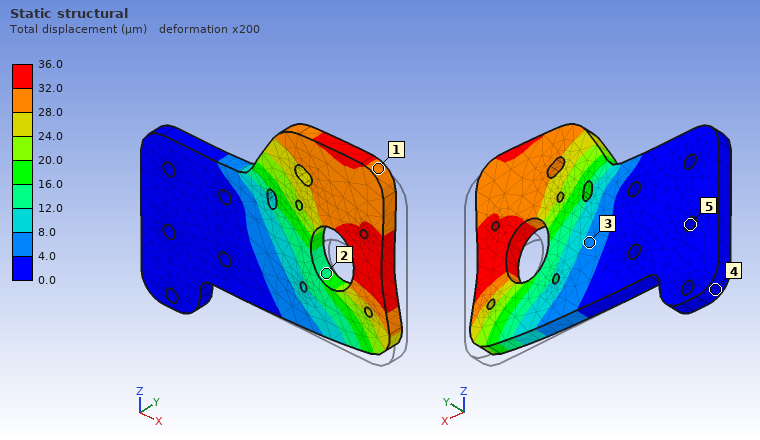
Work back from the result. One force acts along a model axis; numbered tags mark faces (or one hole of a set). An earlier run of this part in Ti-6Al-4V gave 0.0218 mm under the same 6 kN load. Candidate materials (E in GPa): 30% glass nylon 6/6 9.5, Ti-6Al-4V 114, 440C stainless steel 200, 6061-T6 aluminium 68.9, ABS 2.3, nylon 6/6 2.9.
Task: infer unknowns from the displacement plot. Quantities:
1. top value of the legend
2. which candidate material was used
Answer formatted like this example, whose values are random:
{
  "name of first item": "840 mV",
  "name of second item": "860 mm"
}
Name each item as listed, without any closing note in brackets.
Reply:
{
  "top value of the legend": "36.0 µm",
  "which candidate material was used": "6061-T6 aluminium"
}
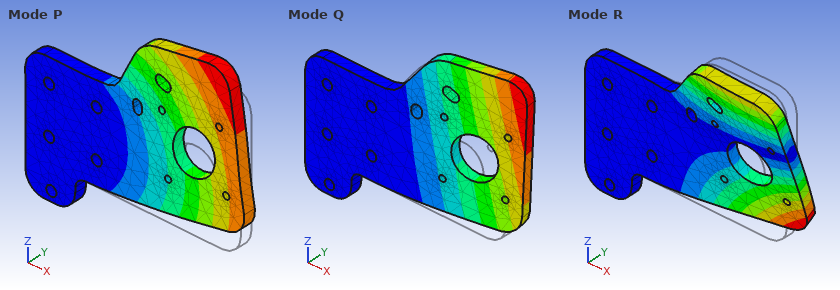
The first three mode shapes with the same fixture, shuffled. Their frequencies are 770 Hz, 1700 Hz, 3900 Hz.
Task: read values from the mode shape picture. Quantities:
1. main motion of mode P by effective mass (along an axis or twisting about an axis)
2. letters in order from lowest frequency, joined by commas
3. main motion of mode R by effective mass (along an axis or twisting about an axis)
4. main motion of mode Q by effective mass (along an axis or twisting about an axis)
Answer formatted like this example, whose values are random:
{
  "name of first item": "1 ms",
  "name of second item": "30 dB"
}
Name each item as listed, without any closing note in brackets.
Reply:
{
  "main motion of mode P by effective mass": "along Z",
  "letters in order from lowest frequency, joined by commas": "Q, R, P",
  "main motion of mode R by effective mass": "twisting about X",
  "main motion of mode Q by effective mass": "along Y"
}
